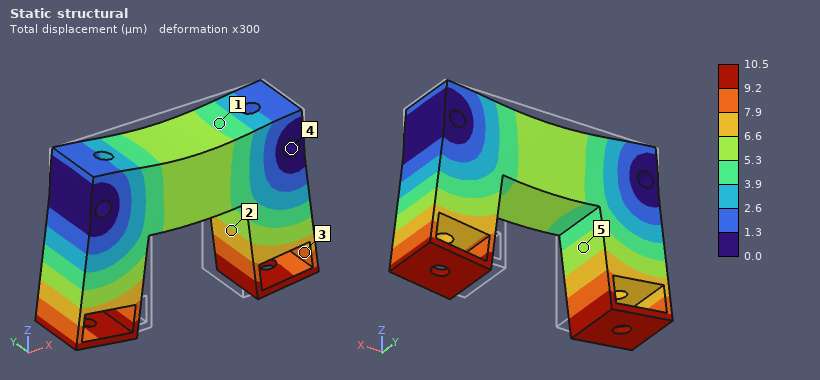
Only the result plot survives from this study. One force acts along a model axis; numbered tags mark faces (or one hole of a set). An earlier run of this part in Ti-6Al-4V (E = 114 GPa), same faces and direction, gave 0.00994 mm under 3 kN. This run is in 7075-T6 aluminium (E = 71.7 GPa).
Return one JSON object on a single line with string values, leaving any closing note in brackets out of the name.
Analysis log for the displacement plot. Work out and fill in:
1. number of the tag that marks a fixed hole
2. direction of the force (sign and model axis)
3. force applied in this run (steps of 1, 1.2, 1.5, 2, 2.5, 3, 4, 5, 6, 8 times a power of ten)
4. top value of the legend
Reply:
{"number of the tag that marks a fixed hole": "4", "direction of the force": "-Z", "force applied in this run": "2 kN", "top value of the legend": "10.5 µm"}
